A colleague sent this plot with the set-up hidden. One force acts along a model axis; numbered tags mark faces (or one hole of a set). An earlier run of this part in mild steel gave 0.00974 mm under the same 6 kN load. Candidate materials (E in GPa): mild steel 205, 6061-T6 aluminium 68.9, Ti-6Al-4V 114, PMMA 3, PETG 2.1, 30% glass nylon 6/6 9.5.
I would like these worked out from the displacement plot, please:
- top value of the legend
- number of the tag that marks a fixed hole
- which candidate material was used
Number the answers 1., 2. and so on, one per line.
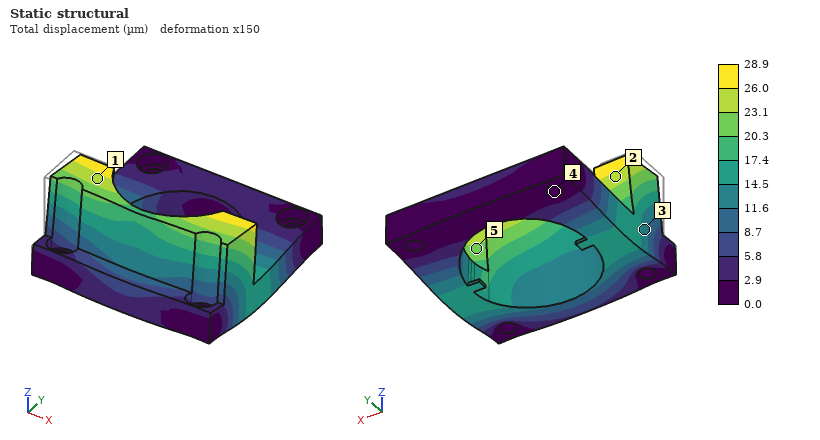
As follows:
1. 28.9 µm
2. 4
3. 6061-T6 aluminium
